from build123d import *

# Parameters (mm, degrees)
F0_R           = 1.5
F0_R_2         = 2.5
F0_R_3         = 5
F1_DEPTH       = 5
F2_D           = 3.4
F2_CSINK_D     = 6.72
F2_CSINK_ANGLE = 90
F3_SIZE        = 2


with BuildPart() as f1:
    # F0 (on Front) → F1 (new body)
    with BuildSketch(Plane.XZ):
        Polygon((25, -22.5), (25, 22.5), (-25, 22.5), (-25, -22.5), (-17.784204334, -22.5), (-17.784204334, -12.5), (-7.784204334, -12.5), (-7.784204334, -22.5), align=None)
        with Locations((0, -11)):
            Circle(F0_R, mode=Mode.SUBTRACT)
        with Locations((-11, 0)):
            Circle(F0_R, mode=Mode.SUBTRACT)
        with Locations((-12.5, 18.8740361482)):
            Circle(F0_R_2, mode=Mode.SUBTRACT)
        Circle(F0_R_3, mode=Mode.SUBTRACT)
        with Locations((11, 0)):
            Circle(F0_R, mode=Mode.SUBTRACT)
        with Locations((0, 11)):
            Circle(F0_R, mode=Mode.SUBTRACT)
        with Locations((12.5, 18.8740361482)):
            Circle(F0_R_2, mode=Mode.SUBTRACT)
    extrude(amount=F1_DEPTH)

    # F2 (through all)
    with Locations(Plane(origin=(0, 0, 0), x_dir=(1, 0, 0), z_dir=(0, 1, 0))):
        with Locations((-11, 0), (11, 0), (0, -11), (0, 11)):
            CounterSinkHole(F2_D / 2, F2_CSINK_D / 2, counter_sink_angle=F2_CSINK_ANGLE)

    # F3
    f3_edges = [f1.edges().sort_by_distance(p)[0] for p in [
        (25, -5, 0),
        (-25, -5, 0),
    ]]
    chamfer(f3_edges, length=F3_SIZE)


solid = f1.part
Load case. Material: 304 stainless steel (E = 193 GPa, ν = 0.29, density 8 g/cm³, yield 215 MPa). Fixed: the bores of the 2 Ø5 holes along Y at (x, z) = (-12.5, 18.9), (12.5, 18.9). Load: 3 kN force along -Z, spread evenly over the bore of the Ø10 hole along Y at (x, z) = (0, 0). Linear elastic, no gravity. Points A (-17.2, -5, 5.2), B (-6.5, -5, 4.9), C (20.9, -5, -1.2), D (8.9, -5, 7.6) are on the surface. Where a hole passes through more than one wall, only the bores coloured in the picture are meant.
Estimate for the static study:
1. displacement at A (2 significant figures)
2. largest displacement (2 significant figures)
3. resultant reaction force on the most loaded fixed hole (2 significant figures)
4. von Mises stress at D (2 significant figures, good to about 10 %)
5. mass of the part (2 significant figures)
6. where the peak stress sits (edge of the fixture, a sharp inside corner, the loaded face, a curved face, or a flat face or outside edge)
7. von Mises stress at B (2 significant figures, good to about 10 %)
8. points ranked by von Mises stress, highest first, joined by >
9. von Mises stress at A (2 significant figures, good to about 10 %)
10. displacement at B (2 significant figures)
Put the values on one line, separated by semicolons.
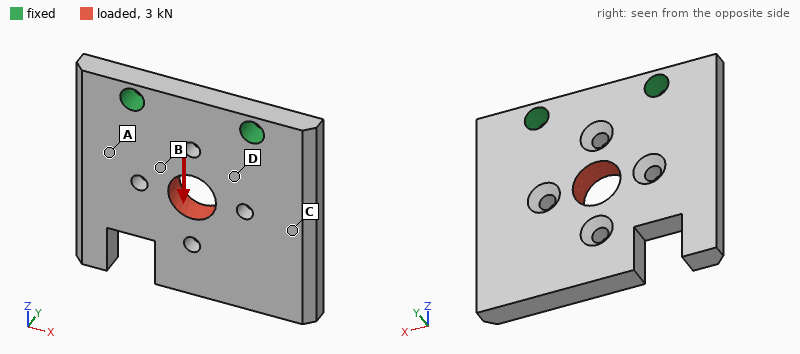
1.0 µm; 3.9 µm; 1.6 kN; 22 MPa; 78 g; a curved face; 27 MPa; B > D > A > C; 8.5 MPa; 1.9 µm
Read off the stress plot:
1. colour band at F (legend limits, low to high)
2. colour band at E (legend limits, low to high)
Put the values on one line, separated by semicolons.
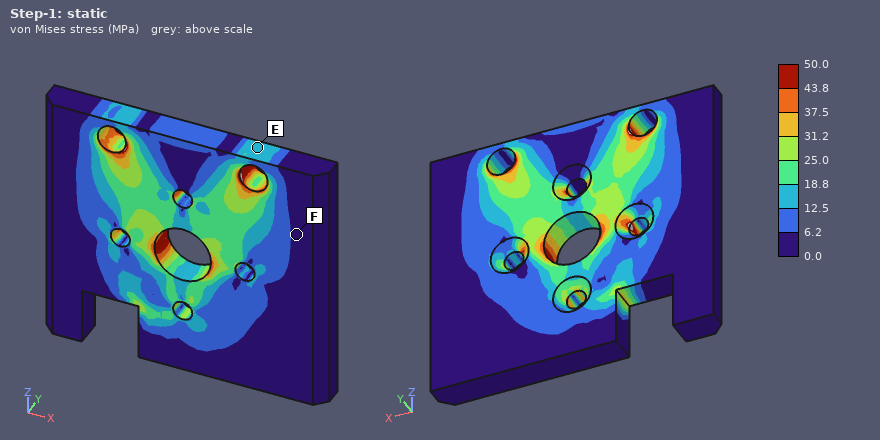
0.0 to 6.2 MPa; 12.5 to 18.8 MPa
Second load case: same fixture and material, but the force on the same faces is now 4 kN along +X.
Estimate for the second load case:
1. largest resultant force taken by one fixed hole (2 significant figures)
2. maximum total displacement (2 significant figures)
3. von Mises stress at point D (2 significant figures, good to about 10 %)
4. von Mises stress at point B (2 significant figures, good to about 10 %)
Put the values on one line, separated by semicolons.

3.1 kN; 21 µm; 41 MPa; 29 MPa
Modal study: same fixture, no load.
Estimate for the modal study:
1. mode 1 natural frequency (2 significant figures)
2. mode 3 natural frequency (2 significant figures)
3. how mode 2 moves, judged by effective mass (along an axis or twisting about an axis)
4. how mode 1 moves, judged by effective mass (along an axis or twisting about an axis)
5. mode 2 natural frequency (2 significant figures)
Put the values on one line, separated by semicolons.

2300 Hz; 9600 Hz; twisting about Z; along Y; 4400 Hz
